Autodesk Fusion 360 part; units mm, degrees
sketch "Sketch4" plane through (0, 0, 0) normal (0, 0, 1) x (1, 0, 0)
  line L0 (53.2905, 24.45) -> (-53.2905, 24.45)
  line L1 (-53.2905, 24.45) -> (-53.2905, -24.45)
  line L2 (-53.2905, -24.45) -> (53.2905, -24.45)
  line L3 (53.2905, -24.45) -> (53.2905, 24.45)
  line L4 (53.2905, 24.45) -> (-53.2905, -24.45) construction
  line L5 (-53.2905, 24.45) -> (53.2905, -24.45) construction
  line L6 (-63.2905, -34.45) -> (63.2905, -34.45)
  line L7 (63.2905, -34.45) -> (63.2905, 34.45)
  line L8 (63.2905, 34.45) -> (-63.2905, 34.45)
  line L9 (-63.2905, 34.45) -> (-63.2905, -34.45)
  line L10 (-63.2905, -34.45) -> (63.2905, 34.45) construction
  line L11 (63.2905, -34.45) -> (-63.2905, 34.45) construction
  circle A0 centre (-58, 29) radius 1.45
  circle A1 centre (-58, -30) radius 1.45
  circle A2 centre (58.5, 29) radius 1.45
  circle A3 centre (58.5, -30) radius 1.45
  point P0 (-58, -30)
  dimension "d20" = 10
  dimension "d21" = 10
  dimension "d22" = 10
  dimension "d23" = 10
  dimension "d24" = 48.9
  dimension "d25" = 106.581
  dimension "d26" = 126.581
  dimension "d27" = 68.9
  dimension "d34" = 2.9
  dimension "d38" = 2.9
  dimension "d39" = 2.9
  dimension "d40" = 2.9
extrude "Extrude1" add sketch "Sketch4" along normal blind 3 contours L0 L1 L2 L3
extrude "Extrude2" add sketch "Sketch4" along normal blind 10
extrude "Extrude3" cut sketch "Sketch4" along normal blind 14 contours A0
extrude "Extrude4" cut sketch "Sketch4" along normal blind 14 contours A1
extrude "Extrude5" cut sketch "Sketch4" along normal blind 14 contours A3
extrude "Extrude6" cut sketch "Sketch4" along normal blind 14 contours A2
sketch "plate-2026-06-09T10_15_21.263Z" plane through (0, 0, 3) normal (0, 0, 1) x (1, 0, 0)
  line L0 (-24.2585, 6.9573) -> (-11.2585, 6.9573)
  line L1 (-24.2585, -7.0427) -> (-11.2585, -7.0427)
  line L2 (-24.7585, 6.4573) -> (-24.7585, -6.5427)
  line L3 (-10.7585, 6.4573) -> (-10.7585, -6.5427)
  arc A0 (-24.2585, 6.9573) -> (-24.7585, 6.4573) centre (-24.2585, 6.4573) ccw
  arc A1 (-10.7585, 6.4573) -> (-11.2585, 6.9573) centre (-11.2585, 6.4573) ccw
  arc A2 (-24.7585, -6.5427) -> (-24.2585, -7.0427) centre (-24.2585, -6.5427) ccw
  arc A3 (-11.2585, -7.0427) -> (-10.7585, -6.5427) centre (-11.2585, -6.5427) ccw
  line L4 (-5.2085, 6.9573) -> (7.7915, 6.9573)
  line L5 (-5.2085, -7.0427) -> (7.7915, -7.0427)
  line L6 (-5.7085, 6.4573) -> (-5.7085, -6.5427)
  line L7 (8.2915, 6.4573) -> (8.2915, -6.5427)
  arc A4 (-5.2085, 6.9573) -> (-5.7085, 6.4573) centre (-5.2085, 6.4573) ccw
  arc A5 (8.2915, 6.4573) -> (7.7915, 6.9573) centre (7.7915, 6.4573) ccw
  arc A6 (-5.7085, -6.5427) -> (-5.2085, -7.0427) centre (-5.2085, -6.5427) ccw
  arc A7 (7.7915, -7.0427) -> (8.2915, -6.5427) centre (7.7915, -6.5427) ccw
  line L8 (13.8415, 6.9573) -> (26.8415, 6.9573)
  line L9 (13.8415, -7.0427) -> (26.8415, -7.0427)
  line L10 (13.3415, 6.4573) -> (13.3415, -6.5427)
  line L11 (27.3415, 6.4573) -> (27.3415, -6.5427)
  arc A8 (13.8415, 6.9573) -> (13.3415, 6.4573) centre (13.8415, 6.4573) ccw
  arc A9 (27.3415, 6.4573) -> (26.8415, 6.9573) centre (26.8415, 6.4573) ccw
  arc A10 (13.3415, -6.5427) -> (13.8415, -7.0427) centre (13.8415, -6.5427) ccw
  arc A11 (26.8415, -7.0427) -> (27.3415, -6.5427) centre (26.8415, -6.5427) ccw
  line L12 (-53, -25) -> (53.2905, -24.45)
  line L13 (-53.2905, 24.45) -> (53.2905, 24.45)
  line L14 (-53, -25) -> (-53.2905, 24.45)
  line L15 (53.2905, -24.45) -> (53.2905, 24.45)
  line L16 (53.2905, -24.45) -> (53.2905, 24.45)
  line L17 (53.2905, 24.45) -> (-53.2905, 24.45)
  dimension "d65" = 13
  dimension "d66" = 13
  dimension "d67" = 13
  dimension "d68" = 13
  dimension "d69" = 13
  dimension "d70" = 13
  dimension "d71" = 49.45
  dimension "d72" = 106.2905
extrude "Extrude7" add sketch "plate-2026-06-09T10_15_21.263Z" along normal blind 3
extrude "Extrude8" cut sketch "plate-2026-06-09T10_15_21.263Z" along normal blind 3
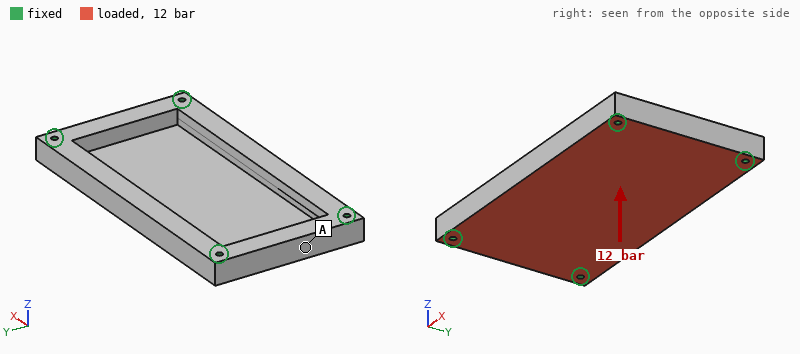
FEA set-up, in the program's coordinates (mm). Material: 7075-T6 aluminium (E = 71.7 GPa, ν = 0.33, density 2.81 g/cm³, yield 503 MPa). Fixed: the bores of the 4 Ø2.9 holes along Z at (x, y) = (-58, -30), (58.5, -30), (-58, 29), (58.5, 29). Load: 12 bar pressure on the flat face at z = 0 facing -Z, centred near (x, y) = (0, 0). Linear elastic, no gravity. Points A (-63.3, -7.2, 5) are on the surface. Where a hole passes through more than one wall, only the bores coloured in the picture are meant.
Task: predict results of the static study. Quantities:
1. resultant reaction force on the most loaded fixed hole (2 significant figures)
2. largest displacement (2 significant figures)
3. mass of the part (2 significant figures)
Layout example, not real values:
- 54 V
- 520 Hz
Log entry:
- 3.1 kN
- 0.51 mm
- 140 g
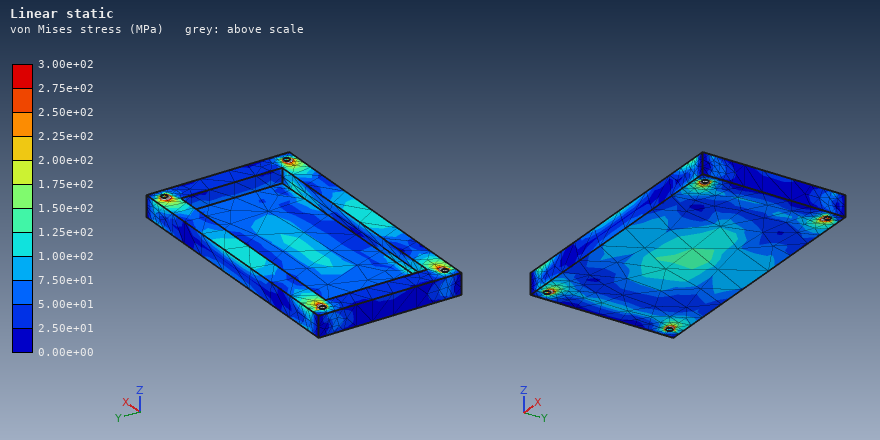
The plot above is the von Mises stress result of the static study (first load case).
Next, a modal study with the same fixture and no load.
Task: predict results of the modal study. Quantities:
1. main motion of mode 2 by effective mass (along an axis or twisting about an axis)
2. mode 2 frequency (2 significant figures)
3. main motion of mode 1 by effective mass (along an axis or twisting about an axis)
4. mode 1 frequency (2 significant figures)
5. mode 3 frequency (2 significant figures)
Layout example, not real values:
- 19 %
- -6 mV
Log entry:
- twisting about X
- 3700 Hz
- along Z
- 2900 Hz
- 5700 Hz
